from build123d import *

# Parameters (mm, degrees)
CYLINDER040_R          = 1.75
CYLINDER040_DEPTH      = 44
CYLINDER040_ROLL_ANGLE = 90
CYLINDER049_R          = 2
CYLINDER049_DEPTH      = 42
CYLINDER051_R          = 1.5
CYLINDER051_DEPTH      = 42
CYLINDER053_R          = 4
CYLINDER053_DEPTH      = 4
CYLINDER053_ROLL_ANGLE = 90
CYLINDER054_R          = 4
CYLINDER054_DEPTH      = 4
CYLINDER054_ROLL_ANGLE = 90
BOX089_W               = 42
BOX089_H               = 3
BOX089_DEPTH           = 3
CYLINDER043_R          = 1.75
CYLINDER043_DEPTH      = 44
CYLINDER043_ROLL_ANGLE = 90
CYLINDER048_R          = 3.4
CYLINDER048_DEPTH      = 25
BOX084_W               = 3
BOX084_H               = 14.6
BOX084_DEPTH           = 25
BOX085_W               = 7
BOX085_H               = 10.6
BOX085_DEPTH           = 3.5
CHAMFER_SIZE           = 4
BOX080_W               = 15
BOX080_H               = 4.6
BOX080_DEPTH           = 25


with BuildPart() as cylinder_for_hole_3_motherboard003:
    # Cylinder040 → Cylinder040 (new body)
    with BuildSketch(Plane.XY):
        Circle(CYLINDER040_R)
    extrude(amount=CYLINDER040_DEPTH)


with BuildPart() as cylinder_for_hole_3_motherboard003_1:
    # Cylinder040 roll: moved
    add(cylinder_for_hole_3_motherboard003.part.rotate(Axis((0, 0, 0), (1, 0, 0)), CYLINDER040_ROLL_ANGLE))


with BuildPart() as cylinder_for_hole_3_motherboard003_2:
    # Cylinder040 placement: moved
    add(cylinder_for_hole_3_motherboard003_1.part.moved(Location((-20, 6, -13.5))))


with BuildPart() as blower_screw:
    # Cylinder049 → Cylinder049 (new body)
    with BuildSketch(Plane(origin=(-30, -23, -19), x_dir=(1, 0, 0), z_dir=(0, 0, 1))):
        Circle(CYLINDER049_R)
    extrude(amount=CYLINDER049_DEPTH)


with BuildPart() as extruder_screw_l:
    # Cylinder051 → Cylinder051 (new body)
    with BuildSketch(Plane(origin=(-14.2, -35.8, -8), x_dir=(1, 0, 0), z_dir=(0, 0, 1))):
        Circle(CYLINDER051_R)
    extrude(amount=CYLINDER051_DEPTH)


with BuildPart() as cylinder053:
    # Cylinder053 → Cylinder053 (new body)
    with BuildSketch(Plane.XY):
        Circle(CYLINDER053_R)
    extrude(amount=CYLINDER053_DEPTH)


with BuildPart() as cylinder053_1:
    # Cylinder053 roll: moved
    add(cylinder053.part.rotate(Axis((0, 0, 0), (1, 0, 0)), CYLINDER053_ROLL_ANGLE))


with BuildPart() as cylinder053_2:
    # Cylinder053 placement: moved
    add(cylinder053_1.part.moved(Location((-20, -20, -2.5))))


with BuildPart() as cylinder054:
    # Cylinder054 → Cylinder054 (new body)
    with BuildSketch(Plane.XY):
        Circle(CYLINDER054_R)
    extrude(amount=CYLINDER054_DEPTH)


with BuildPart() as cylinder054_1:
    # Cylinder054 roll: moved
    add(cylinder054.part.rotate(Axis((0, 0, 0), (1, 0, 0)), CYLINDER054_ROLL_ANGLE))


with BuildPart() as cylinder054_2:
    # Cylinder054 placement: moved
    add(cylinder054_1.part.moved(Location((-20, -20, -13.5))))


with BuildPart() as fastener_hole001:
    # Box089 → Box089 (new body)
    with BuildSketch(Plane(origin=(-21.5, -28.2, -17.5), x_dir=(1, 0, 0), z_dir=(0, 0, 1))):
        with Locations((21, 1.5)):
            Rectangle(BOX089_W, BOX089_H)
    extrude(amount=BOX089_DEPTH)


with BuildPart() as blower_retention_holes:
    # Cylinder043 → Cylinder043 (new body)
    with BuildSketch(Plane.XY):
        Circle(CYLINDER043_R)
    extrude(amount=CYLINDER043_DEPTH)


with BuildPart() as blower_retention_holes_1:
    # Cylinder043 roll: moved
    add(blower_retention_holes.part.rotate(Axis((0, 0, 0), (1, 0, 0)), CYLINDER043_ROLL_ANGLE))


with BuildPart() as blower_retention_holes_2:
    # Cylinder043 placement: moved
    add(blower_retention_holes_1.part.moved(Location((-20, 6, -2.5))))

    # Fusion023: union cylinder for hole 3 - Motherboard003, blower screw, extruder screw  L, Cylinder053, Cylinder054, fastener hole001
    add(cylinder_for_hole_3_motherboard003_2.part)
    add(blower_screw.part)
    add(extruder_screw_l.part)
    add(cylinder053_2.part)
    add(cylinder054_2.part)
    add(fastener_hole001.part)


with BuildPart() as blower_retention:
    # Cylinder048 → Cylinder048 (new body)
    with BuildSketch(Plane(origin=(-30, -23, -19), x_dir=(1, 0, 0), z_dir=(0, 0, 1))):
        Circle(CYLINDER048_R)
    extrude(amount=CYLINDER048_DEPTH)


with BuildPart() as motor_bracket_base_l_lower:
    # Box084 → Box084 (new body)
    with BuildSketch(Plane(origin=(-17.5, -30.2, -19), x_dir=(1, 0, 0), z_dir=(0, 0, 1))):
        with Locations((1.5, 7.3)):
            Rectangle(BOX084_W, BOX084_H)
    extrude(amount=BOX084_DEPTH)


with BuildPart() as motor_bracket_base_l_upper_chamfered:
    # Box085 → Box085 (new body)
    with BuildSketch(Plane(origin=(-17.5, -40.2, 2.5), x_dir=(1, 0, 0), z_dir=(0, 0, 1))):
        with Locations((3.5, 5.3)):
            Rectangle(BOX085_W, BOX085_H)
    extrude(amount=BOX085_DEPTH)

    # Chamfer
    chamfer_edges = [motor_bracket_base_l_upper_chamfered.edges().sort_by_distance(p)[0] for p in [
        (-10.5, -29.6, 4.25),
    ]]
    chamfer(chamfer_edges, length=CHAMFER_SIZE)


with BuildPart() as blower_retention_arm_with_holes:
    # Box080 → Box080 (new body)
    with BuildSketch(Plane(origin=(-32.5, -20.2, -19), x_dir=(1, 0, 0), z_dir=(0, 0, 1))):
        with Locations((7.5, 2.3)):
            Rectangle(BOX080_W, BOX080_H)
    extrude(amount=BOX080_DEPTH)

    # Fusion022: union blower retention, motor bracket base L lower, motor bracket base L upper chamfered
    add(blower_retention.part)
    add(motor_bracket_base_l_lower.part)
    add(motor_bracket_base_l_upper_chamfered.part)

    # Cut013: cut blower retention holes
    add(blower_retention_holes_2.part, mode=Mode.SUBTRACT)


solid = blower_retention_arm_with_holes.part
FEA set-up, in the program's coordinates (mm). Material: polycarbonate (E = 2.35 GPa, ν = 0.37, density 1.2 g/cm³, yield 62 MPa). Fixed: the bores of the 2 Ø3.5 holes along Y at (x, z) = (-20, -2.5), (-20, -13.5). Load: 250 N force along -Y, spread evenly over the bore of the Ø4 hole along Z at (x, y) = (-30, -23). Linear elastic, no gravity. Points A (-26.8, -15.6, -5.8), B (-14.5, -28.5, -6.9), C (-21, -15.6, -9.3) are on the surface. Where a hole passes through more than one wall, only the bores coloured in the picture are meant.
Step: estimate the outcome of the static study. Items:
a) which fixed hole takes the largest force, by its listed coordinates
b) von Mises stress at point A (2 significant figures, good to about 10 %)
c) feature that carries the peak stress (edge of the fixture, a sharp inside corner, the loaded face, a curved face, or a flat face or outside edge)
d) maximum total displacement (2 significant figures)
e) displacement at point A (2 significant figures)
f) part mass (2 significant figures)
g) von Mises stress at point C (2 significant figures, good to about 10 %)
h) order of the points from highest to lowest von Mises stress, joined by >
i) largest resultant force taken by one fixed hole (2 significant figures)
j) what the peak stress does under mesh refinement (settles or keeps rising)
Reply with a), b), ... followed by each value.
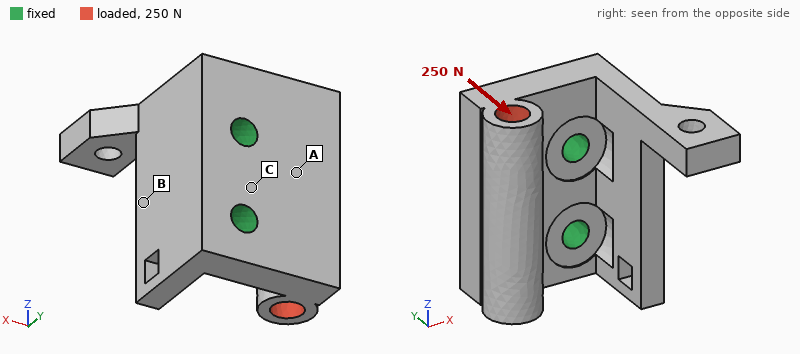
a) (-20, -2.5)
b) 8.2 MPa
c) edge of the fixture
d) 0.35 mm
e) 0.12 mm
f) 4.1 g
g) 12 MPa
h) C > A > B
i) 140 N
j) keeps rising
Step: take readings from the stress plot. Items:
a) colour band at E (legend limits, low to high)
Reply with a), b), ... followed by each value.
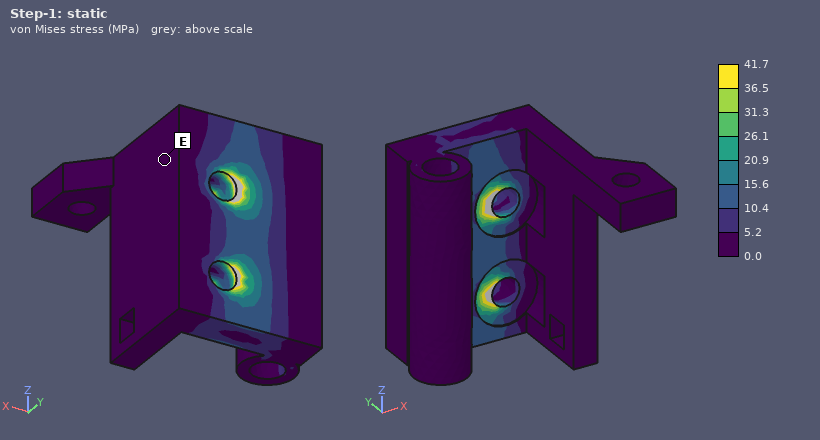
a) 0.0 to 5.2 MPa
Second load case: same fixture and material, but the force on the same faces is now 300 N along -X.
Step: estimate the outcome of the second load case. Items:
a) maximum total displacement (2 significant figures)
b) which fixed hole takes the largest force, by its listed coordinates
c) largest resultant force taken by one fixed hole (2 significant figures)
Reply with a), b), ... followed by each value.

a) 0.45 mm
b) (-20, -2.5)
c) 180 N
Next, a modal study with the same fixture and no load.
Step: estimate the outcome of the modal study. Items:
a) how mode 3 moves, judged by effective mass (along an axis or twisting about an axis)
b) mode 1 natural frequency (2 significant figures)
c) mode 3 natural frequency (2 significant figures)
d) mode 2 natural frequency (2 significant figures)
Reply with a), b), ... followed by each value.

a) along Y
b) 1500 Hz
c) 3900 Hz
d) 3300 Hz
